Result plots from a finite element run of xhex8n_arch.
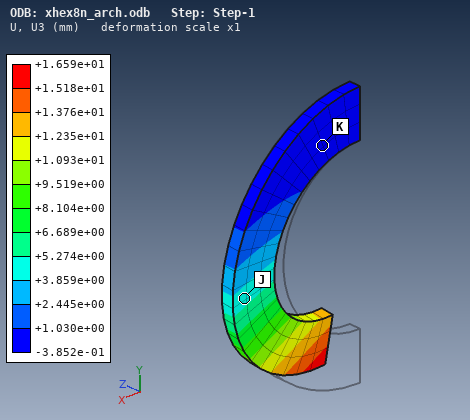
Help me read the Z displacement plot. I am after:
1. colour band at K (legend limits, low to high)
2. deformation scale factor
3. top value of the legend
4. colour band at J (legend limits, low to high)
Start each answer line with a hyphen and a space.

- -3.852e-01 to +1.030e+00 mm
- 1
- +1.659e+01 mm
- +3.859e+00 to +5.274e+00 mm
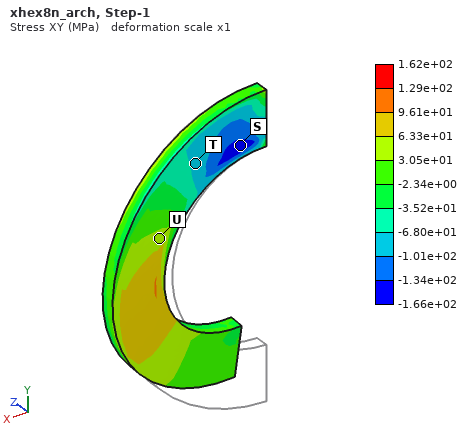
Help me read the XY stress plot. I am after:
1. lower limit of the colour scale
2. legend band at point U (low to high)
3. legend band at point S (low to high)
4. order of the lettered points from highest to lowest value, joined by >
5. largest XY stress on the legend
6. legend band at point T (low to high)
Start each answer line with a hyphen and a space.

- -1.66e+02 MPa
- 3.05e+01 to 6.33e+01 MPa
- -1.66e+02 to -1.34e+02 MPa
- U > T > S
- 1.62e+02 MPa
- -1.01e+02 to -6.80e+01 MPa
